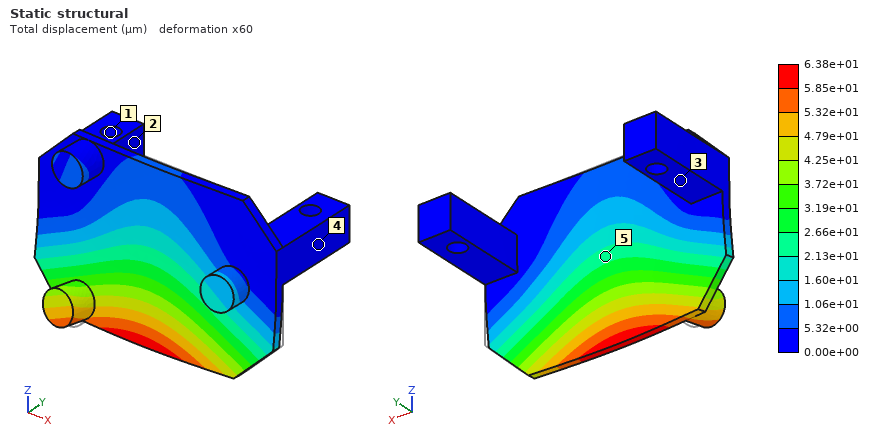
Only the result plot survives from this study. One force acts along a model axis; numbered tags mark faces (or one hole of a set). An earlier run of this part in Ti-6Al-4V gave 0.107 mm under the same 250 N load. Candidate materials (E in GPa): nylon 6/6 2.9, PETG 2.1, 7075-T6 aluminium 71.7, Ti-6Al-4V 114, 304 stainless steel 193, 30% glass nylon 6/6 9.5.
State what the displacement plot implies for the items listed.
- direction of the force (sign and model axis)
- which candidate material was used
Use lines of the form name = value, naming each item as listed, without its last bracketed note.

direction of the force = -Y
which candidate material was used = 304 stainless steel
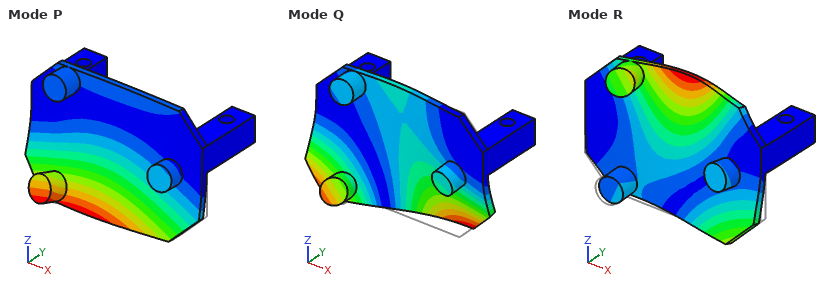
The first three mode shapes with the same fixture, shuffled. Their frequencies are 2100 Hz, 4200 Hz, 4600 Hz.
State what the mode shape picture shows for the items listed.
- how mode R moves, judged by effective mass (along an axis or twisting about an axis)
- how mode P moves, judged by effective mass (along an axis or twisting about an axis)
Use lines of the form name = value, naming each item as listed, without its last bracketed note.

how mode R moves, judged by effective mass = along Y
how mode P moves, judged by effective mass = along Y
